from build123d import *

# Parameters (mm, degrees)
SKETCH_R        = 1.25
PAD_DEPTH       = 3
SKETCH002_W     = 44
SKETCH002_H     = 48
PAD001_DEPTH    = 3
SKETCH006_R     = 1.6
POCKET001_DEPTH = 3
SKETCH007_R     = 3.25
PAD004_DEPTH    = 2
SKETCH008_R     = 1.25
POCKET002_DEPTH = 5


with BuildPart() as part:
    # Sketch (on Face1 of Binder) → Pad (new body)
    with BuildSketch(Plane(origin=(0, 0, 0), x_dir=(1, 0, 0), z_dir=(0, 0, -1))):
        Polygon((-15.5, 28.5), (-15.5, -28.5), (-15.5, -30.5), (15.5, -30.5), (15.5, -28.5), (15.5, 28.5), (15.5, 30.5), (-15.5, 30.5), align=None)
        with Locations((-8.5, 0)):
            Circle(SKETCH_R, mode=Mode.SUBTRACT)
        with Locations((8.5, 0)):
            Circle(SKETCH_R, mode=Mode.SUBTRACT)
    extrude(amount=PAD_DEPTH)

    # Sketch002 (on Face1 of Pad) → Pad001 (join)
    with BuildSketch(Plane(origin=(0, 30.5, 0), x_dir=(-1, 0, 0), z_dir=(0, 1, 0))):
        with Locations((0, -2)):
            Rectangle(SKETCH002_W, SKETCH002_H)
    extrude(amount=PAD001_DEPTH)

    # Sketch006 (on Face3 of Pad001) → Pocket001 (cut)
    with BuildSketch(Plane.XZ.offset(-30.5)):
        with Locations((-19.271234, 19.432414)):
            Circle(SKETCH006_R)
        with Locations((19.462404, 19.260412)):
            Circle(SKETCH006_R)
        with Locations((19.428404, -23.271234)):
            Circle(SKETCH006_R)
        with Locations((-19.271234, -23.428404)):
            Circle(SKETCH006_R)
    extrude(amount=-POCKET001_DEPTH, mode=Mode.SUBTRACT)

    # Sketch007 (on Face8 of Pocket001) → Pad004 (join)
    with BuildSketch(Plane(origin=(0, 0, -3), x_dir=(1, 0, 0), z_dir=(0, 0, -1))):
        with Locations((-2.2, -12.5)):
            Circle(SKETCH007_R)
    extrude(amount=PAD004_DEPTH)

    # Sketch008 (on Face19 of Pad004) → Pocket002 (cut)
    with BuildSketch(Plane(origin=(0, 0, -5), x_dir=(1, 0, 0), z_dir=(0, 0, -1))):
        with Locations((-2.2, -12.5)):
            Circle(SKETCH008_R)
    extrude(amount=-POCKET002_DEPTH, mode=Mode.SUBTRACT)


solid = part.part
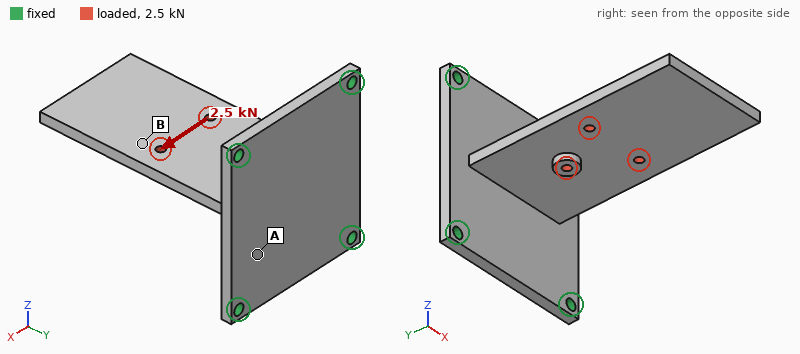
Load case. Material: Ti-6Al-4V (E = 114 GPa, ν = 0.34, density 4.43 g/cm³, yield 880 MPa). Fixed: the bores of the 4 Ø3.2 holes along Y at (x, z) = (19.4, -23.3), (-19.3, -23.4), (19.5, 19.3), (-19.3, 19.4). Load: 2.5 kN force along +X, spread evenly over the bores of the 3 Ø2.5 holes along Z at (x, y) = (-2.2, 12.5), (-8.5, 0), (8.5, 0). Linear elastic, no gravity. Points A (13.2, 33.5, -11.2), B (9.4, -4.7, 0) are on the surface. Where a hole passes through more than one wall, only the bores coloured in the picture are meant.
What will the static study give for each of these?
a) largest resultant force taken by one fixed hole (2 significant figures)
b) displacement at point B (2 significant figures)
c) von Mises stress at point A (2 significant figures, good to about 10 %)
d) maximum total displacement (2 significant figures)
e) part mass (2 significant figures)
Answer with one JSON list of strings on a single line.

["1.2 kN", "0.46 mm", "140 MPa", "0.77 mm", "53 g"]
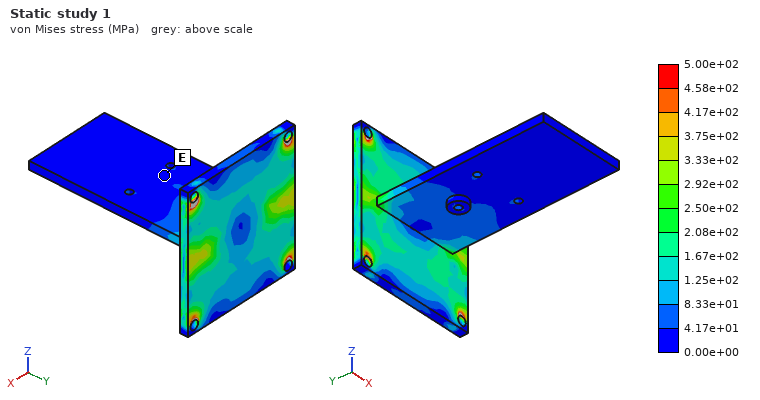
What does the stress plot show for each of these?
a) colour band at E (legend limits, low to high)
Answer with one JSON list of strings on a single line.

["0.00e+00 to 4.17e+01 MPa"]
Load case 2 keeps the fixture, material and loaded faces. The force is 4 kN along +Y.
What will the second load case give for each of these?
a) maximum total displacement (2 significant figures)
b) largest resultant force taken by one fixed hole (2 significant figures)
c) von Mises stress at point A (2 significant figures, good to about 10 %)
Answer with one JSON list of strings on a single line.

["0.36 mm", "1.1 kN", "95 MPa"]
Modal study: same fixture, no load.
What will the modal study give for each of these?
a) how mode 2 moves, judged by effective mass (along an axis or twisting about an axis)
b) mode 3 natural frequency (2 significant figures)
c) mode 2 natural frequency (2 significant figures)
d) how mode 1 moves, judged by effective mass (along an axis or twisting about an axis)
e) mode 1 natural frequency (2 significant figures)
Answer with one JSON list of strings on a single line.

["along X", "2700 Hz", "1900 Hz", "along Z", "620 Hz"]
